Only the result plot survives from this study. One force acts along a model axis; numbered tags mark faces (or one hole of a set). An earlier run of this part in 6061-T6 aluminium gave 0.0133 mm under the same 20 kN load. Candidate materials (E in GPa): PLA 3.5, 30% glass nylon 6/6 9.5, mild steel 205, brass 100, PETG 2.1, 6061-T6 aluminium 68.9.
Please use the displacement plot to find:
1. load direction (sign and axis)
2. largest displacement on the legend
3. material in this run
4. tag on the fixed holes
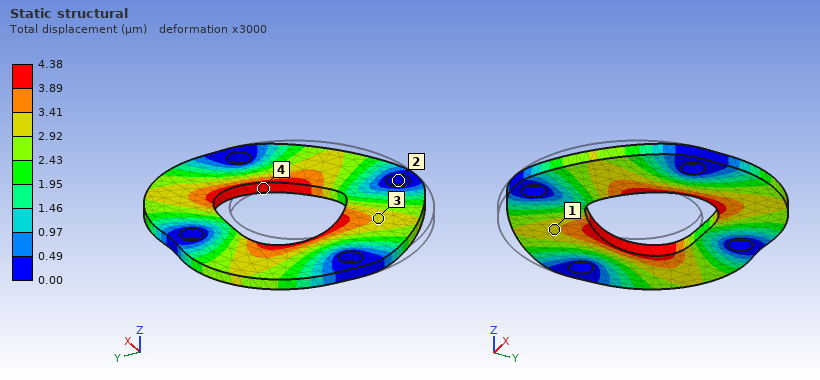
+Y
4.38 µm
mild steel
2
